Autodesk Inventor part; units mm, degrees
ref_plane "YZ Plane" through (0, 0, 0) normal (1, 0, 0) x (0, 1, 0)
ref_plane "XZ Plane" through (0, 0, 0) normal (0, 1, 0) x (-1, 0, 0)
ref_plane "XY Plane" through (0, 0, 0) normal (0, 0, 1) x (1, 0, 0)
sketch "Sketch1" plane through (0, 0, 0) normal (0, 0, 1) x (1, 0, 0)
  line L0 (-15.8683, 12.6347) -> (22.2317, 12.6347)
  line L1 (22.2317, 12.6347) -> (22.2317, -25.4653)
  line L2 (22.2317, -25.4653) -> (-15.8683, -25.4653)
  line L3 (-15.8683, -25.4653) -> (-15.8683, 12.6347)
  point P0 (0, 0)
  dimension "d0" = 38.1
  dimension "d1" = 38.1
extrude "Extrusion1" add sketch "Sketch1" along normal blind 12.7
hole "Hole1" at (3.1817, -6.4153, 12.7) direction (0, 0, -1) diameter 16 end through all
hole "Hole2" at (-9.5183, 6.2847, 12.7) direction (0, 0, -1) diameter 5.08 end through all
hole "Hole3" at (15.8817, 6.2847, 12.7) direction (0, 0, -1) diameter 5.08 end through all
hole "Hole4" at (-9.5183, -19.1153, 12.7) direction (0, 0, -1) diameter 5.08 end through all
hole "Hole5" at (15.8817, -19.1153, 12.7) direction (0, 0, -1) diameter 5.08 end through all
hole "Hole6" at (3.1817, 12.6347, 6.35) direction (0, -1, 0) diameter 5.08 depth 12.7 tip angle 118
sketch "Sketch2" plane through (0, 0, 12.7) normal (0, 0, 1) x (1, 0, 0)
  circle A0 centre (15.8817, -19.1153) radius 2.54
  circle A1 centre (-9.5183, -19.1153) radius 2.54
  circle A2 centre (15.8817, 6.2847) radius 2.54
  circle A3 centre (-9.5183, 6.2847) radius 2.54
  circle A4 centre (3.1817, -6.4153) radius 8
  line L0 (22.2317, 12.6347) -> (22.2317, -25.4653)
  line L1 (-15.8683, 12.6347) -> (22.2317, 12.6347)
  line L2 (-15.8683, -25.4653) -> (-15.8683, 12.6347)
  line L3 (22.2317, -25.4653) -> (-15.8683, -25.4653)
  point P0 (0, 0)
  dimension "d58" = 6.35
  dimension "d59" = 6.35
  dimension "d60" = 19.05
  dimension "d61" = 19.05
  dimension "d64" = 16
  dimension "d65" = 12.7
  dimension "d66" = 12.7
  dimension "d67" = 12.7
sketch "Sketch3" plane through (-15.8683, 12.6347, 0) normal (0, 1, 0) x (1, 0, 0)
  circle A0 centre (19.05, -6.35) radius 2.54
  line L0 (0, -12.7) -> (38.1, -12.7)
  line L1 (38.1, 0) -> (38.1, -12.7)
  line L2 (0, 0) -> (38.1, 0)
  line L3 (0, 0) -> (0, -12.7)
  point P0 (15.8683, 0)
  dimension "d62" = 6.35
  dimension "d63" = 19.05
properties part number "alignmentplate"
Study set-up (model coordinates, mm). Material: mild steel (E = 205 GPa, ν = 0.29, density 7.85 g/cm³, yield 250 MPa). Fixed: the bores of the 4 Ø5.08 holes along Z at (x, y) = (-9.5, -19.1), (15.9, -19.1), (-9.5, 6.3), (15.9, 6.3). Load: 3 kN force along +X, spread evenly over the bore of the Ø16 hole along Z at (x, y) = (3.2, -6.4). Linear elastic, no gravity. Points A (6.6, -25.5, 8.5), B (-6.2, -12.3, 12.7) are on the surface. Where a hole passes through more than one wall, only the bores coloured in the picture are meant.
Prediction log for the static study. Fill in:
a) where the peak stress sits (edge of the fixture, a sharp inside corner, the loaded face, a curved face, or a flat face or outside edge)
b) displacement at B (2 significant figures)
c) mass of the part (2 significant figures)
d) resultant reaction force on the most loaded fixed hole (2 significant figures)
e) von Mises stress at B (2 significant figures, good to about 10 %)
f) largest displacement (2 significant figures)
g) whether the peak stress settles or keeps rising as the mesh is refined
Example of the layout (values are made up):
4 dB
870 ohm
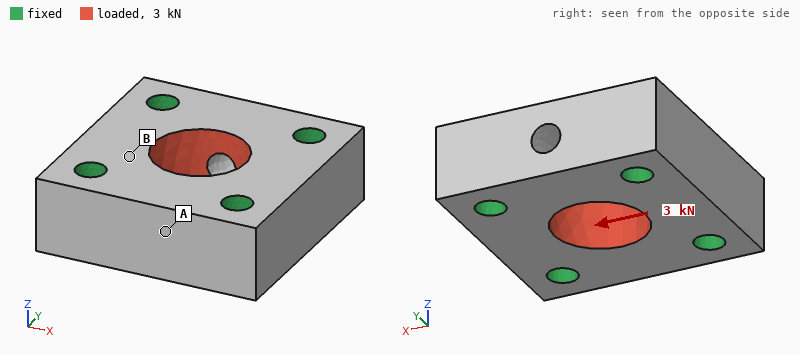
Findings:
edge of the fixture
0.29 µm
110 g
810 N
5.4 MPa
0.52 µm
keeps rising
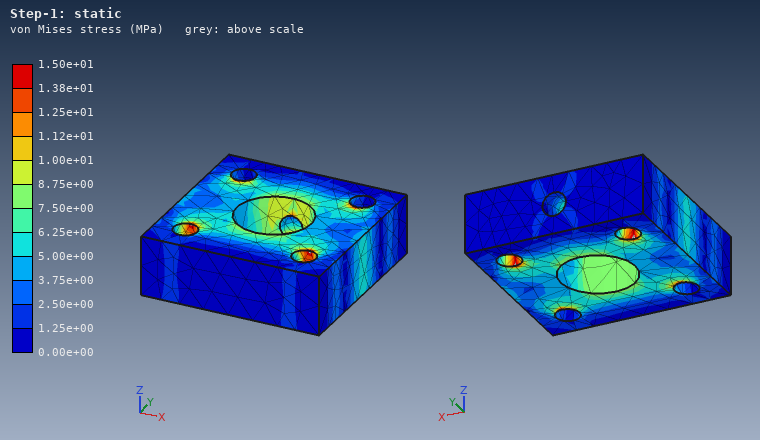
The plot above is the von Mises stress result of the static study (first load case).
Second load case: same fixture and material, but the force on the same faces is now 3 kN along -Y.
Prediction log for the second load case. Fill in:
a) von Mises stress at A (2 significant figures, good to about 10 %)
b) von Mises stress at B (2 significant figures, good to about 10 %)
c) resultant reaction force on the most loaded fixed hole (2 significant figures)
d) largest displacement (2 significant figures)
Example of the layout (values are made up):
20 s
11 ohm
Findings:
4.2 MPa
5.9 MPa
800 N
0.52 µm
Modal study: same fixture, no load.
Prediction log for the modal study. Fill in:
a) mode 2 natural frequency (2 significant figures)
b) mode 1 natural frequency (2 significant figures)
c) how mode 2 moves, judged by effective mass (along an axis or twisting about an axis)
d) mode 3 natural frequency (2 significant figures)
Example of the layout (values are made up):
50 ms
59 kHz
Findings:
55 kHz
48 kHz
along Z
58 kHz
